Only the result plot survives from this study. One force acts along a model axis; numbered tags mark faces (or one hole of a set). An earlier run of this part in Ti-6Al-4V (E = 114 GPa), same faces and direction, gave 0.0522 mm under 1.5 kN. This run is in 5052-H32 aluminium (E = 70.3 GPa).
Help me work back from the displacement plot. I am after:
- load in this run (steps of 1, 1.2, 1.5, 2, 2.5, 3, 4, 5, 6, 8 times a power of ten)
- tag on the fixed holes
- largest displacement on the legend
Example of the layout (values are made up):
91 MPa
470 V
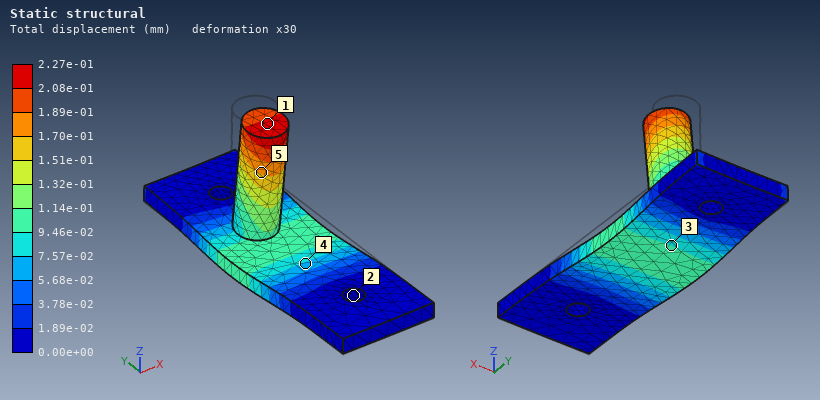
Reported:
4 kN
2
2.27e-01 mm
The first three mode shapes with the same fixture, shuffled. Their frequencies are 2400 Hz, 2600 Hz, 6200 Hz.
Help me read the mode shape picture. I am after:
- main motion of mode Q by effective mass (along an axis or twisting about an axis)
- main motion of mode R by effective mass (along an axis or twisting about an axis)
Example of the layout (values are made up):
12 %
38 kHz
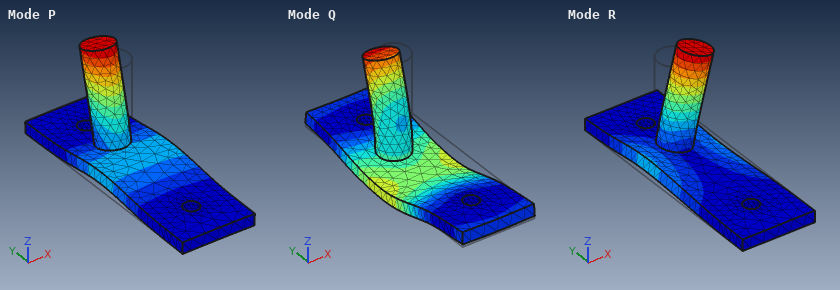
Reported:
along Z
along X
